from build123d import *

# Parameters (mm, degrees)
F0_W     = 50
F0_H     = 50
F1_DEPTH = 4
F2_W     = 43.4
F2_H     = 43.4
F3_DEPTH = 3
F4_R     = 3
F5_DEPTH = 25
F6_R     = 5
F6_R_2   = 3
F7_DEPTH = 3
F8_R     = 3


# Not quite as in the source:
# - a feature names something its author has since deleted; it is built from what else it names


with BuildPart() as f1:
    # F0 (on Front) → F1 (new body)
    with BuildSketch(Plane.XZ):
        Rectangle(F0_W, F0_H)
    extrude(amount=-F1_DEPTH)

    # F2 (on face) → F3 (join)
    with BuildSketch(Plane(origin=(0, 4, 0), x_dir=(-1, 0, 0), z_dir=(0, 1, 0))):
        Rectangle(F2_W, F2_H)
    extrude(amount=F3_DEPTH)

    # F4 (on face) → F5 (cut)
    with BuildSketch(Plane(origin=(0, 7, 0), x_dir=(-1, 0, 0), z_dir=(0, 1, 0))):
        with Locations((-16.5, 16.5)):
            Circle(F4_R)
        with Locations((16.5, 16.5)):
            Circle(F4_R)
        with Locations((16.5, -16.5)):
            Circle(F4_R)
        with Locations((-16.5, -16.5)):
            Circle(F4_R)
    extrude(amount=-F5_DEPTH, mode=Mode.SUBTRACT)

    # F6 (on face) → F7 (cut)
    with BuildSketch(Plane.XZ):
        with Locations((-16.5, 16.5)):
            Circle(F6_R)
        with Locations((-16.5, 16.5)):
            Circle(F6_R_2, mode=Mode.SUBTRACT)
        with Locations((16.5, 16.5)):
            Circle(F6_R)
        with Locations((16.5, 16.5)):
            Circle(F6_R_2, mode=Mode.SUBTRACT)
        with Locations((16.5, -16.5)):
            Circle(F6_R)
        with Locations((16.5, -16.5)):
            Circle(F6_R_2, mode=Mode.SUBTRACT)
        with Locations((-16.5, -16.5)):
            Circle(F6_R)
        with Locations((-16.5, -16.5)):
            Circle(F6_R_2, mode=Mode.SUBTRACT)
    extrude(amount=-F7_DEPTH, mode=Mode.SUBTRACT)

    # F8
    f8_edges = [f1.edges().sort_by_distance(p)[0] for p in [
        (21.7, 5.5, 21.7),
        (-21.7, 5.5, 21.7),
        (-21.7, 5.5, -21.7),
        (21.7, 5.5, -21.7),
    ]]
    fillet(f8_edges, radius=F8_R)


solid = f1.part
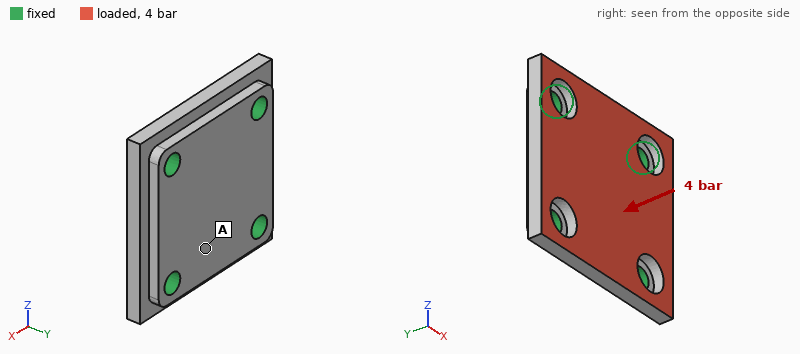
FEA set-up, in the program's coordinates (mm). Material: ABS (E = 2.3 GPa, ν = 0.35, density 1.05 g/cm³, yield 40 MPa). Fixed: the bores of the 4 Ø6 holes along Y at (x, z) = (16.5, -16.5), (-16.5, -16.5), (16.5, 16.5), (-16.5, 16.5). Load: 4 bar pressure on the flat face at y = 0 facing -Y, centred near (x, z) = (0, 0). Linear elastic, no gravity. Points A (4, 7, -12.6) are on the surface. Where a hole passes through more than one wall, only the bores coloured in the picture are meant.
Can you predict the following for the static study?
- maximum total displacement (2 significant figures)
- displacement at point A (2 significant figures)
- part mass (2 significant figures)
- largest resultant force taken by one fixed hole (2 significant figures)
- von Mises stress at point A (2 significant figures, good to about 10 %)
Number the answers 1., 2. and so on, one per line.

1. 59 µm
2. 43 µm
3. 15 g
4. 230 N
5. 2.0 MPa
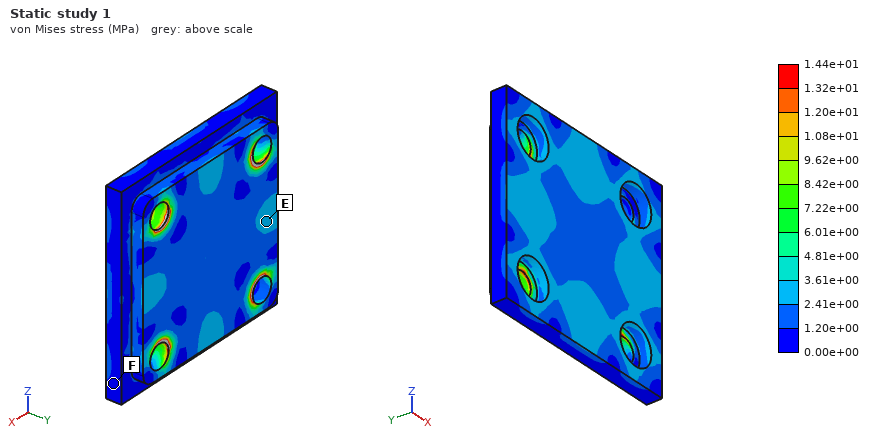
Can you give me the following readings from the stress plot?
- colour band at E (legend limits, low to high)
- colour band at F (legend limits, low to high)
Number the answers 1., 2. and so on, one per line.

1. 2.41e+00 to 3.61e+00 MPa
2. 0.00e+00 to 1.20e+00 MPa
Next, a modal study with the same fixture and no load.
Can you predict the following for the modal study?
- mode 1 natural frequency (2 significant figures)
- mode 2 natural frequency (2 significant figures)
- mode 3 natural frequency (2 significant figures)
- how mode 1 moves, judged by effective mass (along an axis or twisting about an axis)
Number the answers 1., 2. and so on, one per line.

1. 5500 Hz
2. 7200 Hz
3. 7400 Hz
4. along Y
